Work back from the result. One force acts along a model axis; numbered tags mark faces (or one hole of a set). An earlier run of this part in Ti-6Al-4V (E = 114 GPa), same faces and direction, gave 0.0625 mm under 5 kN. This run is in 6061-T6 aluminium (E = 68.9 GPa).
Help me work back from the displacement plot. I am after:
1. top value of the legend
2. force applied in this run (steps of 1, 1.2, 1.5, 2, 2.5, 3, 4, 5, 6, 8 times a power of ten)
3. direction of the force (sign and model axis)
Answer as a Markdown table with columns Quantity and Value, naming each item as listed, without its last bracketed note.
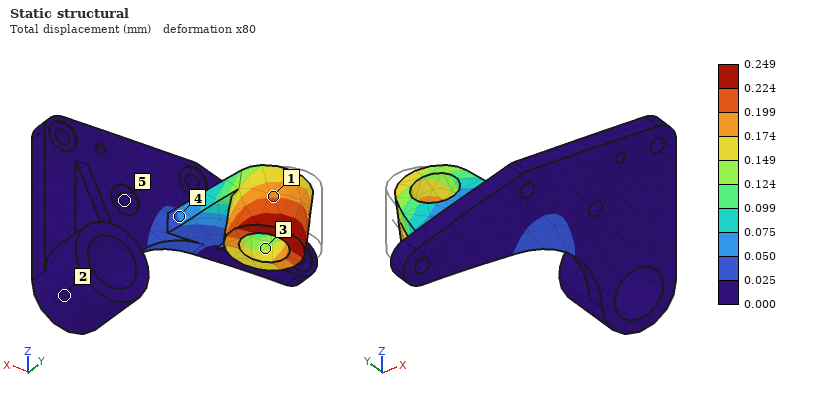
| Quantity | Value |
|---|---|
| top value of the legend | 0.249 mm |
| force applied in this run | 12 kN |
| direction of the force | +X |
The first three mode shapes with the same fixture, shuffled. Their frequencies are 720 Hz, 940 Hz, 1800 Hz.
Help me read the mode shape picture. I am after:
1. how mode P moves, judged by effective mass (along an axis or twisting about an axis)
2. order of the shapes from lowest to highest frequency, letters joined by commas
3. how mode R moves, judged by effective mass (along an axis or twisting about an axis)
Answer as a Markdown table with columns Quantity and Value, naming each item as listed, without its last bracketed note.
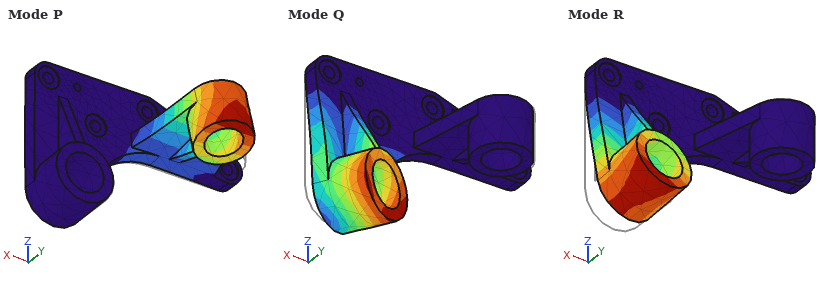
| Quantity | Value |
|---|---|
| how mode P moves, judged by effective mass | along Z |
| order of the shapes from lowest to highest frequency, letters joined by commas | R, P, Q |
| how mode R moves, judged by effective mass | along Y |
